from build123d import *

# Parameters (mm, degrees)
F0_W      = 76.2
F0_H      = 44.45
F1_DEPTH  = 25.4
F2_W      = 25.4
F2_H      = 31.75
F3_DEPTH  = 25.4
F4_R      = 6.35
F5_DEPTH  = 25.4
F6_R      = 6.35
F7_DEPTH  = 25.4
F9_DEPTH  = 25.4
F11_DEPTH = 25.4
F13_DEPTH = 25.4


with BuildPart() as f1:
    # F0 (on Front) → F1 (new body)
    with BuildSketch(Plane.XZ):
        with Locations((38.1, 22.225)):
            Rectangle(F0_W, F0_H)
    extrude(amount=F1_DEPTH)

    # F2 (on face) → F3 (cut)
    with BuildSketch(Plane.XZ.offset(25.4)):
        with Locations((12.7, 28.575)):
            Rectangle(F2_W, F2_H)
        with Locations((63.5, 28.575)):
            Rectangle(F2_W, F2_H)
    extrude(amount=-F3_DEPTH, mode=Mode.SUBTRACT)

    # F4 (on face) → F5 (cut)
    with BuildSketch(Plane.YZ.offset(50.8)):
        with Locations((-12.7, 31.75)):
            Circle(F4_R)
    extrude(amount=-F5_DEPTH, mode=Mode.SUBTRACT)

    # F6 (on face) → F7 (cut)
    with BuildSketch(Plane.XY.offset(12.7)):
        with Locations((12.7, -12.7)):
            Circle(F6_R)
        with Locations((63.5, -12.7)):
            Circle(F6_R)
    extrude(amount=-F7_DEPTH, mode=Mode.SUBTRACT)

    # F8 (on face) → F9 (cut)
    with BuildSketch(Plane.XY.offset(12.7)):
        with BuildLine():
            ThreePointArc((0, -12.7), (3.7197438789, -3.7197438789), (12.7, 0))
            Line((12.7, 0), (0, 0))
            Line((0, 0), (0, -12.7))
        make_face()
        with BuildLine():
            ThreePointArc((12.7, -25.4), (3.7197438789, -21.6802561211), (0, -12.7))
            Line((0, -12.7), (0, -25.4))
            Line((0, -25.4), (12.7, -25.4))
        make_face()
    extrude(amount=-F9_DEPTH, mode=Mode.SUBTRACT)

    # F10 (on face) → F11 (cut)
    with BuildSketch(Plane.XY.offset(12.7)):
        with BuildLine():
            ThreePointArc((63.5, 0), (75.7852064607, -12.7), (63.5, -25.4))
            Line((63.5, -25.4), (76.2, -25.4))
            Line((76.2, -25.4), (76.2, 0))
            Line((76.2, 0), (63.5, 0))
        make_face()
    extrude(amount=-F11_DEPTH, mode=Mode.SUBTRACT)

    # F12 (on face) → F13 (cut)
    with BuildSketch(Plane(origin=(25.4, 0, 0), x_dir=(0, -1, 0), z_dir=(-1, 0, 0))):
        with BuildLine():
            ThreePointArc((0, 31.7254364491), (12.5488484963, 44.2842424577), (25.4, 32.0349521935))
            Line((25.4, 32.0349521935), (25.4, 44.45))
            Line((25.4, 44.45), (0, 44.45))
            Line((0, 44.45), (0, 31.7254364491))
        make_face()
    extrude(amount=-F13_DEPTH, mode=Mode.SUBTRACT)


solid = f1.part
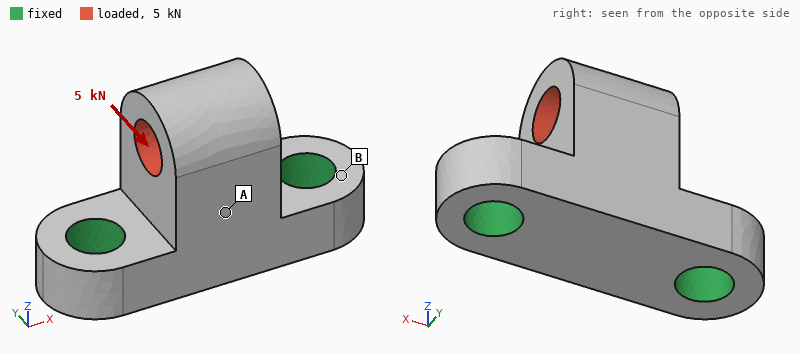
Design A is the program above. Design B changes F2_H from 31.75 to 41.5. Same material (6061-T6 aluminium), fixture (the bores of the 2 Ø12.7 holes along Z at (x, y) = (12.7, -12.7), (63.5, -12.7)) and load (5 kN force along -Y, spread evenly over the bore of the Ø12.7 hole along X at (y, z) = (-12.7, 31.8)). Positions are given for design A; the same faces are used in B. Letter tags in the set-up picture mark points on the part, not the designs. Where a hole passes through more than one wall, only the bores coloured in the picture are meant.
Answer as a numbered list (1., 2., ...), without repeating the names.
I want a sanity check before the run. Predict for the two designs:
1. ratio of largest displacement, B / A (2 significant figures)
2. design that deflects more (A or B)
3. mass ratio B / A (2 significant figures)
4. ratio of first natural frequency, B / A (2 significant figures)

1. 2.4
2. B
3. 0.88
4. 0.62
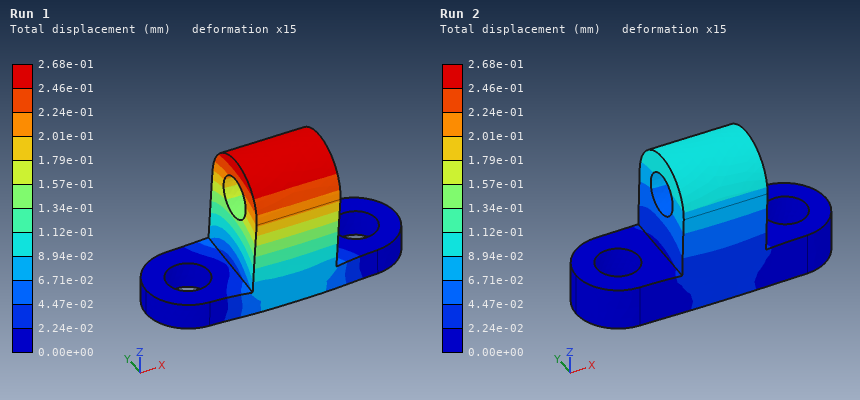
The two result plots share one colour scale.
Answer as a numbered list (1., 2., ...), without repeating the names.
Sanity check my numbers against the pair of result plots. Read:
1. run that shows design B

1. Run 1
